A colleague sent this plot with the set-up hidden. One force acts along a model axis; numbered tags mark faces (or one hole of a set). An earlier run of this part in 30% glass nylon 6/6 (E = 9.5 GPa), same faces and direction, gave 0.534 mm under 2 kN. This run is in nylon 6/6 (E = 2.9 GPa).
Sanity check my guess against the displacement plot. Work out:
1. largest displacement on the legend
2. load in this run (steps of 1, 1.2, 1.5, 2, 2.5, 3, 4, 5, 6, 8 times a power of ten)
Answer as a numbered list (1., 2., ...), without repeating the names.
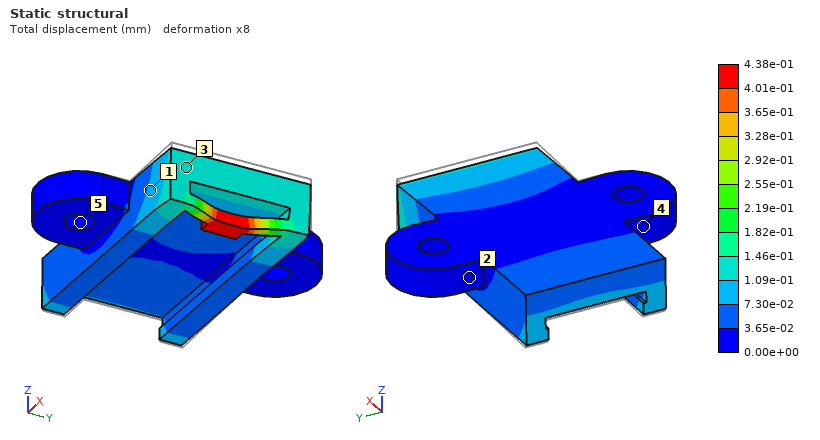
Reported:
1. 4.38e-01 mm
2. 500 N
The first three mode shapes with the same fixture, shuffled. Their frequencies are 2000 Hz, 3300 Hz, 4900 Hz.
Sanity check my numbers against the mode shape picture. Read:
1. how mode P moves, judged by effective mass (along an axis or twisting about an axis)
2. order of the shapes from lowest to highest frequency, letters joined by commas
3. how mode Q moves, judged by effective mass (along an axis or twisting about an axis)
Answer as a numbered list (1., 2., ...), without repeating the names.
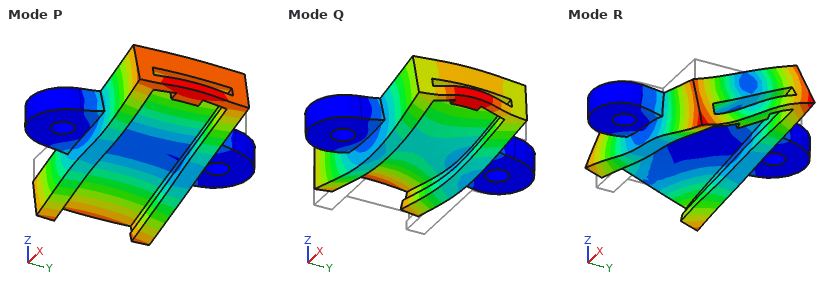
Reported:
1. twisting about Y
2. P, Q, R
3. along Z
